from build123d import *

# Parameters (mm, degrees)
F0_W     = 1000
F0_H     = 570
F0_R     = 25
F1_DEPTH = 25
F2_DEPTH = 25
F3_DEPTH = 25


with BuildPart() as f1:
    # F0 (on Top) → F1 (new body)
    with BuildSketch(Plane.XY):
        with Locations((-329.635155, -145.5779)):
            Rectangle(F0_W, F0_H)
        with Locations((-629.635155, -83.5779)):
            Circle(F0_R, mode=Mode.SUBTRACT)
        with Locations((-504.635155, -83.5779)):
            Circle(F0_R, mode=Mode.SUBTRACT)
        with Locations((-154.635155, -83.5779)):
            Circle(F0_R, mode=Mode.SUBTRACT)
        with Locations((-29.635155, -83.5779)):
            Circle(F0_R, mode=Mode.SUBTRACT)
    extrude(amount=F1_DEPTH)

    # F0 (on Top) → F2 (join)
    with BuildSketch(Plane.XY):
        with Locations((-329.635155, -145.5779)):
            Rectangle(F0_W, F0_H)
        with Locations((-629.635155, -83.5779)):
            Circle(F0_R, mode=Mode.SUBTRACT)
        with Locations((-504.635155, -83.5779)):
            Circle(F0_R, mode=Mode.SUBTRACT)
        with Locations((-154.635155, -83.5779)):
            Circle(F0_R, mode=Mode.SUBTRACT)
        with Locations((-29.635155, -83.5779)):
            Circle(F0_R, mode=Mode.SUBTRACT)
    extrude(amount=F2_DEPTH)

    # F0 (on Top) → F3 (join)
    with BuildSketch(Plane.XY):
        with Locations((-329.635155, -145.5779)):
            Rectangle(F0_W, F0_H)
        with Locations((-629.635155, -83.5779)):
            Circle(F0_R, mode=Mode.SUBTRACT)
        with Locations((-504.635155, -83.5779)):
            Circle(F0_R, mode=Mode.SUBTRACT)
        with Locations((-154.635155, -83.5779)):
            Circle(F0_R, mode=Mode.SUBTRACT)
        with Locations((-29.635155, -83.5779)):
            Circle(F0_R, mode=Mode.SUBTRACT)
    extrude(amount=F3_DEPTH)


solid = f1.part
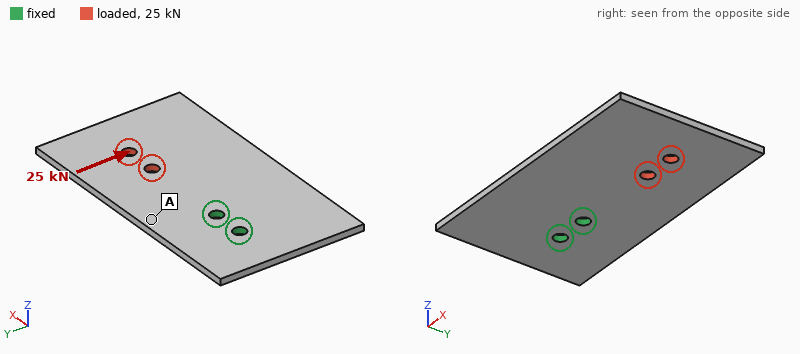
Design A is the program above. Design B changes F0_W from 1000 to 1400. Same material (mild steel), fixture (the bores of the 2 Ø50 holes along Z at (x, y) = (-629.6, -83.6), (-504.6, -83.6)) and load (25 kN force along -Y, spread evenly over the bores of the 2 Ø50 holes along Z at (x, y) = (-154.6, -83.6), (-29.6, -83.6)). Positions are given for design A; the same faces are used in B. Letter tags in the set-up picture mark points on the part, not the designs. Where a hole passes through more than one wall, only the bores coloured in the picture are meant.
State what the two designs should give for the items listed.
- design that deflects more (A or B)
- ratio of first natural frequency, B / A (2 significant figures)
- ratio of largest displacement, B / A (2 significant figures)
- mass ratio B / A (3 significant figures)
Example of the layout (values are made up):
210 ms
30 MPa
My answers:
B
0.60
1.2
1.41
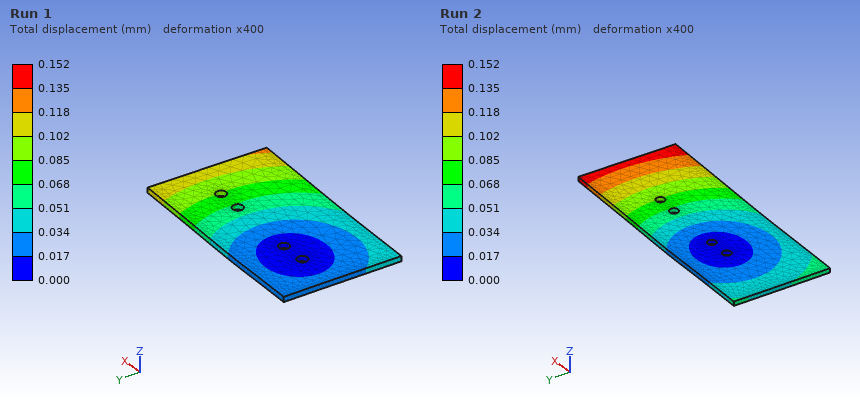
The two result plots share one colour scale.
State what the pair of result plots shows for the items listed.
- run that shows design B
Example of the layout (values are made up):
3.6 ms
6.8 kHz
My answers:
Run 2
